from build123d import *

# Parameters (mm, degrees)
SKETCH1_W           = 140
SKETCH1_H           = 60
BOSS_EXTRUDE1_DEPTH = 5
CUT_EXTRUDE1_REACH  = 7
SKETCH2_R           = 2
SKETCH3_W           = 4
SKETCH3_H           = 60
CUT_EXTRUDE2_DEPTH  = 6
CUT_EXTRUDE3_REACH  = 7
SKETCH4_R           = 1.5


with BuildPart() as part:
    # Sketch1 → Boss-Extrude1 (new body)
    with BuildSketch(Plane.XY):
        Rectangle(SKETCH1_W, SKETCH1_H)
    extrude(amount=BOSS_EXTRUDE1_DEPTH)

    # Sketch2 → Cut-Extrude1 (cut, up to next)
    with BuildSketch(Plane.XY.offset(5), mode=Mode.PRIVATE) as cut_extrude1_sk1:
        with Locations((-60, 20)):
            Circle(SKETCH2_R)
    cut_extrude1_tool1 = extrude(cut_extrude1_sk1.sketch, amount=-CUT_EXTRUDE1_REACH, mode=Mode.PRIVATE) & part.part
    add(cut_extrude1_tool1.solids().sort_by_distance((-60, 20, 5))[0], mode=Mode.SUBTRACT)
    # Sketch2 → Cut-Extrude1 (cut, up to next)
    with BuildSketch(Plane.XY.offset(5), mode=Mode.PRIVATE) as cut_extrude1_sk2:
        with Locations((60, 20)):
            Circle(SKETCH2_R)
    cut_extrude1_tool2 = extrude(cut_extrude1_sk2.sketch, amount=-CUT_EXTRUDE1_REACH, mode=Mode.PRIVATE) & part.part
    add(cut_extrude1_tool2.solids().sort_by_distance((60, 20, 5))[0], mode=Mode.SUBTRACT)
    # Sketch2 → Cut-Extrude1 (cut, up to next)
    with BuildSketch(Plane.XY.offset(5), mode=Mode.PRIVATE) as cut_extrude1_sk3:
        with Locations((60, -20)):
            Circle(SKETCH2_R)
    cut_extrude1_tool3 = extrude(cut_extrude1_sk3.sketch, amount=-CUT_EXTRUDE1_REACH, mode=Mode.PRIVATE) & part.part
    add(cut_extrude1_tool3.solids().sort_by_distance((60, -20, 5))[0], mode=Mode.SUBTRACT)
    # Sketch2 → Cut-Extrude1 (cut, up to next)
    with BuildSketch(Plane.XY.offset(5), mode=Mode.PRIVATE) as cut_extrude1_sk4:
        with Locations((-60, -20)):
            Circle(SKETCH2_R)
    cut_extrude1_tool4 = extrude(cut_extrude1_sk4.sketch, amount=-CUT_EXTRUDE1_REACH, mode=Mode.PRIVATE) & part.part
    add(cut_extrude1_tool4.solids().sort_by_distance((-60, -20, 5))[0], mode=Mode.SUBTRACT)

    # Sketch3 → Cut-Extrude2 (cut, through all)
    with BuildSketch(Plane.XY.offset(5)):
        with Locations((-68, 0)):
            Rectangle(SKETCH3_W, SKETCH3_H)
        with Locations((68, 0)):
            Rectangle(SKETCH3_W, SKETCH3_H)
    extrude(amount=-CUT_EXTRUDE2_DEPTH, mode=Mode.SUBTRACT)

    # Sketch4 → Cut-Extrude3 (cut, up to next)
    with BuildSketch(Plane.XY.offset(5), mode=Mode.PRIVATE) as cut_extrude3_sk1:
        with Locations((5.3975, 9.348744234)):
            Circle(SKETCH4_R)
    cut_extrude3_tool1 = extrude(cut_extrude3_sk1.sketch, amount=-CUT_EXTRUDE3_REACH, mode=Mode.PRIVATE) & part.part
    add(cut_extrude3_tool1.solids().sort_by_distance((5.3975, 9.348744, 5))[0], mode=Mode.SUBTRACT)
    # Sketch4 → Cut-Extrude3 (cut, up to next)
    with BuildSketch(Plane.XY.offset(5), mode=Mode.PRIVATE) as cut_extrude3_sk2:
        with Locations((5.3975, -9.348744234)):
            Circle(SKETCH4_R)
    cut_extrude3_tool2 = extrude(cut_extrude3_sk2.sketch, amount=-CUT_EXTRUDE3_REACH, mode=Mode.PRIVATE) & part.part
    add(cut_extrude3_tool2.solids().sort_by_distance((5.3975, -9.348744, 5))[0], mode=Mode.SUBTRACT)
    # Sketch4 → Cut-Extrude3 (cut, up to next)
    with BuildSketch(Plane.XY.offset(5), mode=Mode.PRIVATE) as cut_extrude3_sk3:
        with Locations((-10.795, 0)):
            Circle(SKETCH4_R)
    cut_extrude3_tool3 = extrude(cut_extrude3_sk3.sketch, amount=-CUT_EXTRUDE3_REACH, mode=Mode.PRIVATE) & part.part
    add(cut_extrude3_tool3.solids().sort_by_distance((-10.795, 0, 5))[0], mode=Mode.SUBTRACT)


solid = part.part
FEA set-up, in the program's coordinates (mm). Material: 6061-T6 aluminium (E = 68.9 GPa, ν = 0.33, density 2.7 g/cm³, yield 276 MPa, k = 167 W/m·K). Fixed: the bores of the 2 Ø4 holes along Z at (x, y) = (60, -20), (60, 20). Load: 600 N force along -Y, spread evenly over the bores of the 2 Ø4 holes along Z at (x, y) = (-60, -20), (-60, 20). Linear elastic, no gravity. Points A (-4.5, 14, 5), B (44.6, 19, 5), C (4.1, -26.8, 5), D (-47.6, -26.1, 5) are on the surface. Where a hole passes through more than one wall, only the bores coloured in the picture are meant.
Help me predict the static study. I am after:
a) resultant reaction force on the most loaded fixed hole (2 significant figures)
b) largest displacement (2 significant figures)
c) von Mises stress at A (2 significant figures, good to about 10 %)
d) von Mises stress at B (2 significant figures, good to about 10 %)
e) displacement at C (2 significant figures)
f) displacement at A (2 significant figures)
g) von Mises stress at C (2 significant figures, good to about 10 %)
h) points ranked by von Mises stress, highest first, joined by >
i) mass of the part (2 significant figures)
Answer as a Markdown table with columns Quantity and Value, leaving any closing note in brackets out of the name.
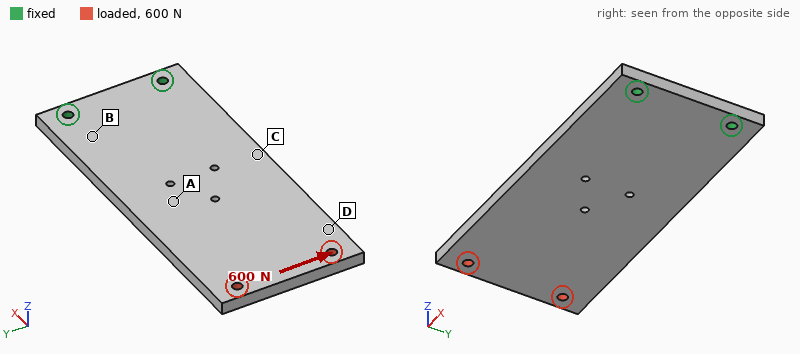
| Quantity | Value |
|---|---|
| resultant reaction force on the most loaded fixed hole | 1.7 kN |
| largest displacement | 86 µm |
| von Mises stress at A | 6.9 MPa |
| von Mises stress at B | 16 MPa |
| displacement at C | 31 µm |
| displacement at A | 33 µm |
| von Mises stress at C | 12 MPa |
| points ranked by von Mises stress, highest first, joined by > | B > C > A > D |
| mass of the part | 110 g |
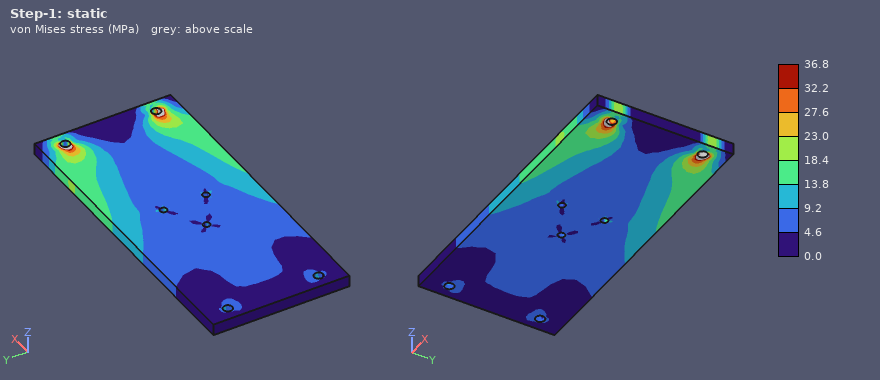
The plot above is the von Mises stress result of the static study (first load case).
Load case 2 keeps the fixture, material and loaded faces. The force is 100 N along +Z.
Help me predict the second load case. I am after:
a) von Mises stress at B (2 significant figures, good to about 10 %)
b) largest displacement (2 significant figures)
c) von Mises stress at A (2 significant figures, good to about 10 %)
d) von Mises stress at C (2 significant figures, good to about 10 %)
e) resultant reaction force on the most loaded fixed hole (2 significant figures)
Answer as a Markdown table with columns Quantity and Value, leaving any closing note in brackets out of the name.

| Quantity | Value |
|---|---|
| von Mises stress at B | 40 MPa |
| largest displacement | 1.5 mm |
| von Mises stress at A | 22 MPa |
| von Mises stress at C | 27 MPa |
| resultant reaction force on the most loaded fixed hole | 50 N |
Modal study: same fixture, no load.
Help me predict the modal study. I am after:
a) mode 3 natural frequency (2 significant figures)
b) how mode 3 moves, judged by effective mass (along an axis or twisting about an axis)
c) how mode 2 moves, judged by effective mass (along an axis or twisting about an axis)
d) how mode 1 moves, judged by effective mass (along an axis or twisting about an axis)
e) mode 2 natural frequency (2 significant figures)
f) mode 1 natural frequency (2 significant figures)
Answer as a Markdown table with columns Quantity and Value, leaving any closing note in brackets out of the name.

| Quantity | Value |
|---|---|
| mode 3 natural frequency | 1600 Hz |
| how mode 3 moves, judged by effective mass | along Z |
| how mode 2 moves, judged by effective mass | twisting about X |
| how mode 1 moves, judged by effective mass | along Z |
| mode 2 natural frequency | 1100 Hz |
| mode 1 natural frequency | 250 Hz |
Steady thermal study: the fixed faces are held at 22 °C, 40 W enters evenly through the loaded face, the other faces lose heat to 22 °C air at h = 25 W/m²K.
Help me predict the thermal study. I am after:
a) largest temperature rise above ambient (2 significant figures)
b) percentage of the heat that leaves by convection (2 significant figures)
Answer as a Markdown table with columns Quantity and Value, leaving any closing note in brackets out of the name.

| Quantity | Value |
|---|---|
| largest temperature rise above ambient | 79 K |
| percentage of the heat that leaves by convection | 39 % |
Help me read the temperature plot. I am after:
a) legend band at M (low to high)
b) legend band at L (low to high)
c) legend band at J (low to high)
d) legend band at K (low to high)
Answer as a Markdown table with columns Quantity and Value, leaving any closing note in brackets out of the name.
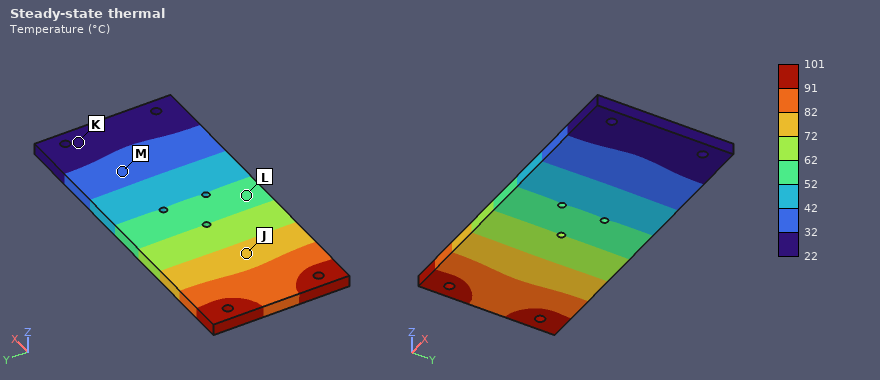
| Quantity | Value |
|---|---|
| legend band at M | 32 to 42 °C |
| legend band at L | 52 to 62 °C |
| legend band at J | 72 to 82 °C |
| legend band at K | 22 to 32 °C |
